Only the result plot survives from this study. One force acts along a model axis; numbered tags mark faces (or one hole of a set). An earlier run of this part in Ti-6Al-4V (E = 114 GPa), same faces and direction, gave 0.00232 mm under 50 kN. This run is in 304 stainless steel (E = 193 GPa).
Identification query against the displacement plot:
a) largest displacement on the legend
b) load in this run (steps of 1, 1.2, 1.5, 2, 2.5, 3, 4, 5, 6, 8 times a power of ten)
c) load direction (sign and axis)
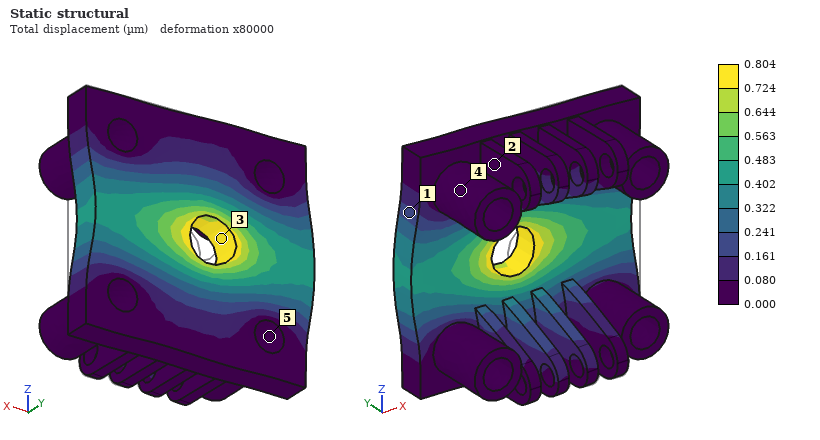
0.804 µm
30 kN
-X
